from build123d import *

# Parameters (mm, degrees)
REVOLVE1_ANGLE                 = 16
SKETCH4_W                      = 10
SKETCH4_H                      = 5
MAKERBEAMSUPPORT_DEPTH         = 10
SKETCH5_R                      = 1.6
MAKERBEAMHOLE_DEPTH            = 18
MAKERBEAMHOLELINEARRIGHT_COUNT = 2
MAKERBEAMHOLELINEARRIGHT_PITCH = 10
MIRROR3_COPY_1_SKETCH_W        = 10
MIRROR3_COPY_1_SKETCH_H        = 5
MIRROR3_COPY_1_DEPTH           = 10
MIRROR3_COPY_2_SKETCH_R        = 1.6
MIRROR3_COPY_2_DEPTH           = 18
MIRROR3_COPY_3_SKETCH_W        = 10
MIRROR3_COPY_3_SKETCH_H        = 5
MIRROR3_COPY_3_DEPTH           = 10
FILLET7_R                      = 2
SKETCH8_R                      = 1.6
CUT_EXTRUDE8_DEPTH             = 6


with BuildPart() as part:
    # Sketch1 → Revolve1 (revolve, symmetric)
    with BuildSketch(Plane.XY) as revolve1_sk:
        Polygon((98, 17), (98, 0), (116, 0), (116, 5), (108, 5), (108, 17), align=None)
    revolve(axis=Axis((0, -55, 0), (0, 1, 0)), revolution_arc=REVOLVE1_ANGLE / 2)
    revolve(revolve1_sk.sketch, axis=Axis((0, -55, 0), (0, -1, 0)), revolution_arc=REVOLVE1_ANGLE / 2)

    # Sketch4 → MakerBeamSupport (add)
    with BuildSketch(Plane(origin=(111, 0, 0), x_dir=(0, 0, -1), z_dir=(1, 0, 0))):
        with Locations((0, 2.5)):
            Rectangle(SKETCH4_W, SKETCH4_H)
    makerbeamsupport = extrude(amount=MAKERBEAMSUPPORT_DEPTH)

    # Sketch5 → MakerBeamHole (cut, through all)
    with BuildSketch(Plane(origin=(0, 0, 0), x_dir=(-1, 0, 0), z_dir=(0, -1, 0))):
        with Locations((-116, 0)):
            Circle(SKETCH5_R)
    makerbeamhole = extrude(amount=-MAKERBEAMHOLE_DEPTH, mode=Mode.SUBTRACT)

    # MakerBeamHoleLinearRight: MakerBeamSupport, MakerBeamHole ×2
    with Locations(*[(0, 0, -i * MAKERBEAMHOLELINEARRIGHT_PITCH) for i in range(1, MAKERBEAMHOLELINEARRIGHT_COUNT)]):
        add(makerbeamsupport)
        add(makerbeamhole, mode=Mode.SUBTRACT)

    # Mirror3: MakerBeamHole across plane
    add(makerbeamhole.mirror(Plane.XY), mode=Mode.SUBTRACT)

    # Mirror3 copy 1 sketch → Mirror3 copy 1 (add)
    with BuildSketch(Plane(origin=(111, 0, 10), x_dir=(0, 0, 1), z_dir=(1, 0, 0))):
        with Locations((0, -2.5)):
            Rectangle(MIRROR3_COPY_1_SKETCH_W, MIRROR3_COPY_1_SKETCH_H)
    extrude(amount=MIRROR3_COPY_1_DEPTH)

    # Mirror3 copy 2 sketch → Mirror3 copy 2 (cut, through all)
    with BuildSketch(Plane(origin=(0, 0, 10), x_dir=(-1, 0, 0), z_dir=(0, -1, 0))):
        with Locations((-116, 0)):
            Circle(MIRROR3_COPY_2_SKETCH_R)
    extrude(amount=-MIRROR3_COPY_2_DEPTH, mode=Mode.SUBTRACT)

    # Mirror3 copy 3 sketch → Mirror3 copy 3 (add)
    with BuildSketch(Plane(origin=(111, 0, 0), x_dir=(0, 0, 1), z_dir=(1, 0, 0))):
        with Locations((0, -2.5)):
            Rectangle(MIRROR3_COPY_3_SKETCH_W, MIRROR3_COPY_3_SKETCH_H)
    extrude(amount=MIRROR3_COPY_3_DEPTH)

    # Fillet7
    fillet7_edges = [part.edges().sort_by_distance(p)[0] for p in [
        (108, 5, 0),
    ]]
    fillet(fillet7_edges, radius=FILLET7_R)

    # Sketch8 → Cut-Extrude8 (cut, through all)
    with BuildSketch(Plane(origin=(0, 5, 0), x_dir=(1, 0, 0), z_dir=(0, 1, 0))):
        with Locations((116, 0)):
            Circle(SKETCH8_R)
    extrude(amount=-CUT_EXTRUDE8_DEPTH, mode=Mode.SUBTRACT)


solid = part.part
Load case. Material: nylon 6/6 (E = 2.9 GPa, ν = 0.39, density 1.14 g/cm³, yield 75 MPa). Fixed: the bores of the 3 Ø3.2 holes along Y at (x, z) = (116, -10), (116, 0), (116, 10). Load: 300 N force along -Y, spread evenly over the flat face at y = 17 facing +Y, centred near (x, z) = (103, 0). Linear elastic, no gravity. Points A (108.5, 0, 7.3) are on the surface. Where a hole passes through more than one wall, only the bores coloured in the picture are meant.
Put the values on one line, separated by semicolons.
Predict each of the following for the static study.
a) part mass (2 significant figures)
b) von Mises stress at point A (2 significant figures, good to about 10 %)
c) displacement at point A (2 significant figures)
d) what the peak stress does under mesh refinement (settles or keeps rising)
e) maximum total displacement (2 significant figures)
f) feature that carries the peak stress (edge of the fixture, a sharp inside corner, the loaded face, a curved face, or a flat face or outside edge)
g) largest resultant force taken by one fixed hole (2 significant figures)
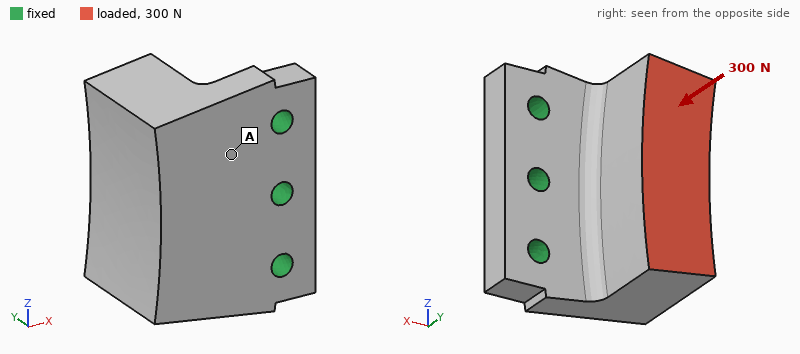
7.8 g; 11 MPa; 0.11 mm; keeps rising; 0.51 mm; edge of the fixture; 110 N
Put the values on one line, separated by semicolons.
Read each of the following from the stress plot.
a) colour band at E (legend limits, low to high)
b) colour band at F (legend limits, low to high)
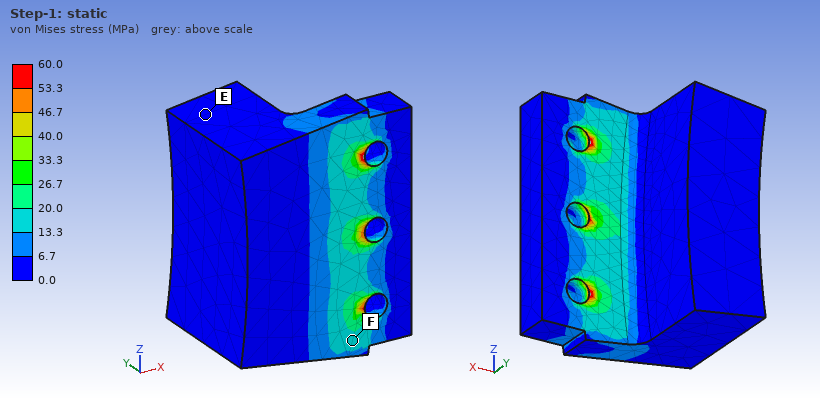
0.0 to 6.7 MPa; 13.3 to 20.0 MPa
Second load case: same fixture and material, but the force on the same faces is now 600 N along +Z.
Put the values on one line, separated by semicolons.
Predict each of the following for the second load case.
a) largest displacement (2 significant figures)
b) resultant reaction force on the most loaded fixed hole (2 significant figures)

0.44 mm; 540 N
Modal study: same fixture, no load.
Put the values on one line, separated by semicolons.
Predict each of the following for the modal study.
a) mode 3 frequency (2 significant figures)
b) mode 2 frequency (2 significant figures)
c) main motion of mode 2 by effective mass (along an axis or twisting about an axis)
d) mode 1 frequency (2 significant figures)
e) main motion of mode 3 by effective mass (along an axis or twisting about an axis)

6400 Hz; 3800 Hz; along Z; 1800 Hz; along Z
